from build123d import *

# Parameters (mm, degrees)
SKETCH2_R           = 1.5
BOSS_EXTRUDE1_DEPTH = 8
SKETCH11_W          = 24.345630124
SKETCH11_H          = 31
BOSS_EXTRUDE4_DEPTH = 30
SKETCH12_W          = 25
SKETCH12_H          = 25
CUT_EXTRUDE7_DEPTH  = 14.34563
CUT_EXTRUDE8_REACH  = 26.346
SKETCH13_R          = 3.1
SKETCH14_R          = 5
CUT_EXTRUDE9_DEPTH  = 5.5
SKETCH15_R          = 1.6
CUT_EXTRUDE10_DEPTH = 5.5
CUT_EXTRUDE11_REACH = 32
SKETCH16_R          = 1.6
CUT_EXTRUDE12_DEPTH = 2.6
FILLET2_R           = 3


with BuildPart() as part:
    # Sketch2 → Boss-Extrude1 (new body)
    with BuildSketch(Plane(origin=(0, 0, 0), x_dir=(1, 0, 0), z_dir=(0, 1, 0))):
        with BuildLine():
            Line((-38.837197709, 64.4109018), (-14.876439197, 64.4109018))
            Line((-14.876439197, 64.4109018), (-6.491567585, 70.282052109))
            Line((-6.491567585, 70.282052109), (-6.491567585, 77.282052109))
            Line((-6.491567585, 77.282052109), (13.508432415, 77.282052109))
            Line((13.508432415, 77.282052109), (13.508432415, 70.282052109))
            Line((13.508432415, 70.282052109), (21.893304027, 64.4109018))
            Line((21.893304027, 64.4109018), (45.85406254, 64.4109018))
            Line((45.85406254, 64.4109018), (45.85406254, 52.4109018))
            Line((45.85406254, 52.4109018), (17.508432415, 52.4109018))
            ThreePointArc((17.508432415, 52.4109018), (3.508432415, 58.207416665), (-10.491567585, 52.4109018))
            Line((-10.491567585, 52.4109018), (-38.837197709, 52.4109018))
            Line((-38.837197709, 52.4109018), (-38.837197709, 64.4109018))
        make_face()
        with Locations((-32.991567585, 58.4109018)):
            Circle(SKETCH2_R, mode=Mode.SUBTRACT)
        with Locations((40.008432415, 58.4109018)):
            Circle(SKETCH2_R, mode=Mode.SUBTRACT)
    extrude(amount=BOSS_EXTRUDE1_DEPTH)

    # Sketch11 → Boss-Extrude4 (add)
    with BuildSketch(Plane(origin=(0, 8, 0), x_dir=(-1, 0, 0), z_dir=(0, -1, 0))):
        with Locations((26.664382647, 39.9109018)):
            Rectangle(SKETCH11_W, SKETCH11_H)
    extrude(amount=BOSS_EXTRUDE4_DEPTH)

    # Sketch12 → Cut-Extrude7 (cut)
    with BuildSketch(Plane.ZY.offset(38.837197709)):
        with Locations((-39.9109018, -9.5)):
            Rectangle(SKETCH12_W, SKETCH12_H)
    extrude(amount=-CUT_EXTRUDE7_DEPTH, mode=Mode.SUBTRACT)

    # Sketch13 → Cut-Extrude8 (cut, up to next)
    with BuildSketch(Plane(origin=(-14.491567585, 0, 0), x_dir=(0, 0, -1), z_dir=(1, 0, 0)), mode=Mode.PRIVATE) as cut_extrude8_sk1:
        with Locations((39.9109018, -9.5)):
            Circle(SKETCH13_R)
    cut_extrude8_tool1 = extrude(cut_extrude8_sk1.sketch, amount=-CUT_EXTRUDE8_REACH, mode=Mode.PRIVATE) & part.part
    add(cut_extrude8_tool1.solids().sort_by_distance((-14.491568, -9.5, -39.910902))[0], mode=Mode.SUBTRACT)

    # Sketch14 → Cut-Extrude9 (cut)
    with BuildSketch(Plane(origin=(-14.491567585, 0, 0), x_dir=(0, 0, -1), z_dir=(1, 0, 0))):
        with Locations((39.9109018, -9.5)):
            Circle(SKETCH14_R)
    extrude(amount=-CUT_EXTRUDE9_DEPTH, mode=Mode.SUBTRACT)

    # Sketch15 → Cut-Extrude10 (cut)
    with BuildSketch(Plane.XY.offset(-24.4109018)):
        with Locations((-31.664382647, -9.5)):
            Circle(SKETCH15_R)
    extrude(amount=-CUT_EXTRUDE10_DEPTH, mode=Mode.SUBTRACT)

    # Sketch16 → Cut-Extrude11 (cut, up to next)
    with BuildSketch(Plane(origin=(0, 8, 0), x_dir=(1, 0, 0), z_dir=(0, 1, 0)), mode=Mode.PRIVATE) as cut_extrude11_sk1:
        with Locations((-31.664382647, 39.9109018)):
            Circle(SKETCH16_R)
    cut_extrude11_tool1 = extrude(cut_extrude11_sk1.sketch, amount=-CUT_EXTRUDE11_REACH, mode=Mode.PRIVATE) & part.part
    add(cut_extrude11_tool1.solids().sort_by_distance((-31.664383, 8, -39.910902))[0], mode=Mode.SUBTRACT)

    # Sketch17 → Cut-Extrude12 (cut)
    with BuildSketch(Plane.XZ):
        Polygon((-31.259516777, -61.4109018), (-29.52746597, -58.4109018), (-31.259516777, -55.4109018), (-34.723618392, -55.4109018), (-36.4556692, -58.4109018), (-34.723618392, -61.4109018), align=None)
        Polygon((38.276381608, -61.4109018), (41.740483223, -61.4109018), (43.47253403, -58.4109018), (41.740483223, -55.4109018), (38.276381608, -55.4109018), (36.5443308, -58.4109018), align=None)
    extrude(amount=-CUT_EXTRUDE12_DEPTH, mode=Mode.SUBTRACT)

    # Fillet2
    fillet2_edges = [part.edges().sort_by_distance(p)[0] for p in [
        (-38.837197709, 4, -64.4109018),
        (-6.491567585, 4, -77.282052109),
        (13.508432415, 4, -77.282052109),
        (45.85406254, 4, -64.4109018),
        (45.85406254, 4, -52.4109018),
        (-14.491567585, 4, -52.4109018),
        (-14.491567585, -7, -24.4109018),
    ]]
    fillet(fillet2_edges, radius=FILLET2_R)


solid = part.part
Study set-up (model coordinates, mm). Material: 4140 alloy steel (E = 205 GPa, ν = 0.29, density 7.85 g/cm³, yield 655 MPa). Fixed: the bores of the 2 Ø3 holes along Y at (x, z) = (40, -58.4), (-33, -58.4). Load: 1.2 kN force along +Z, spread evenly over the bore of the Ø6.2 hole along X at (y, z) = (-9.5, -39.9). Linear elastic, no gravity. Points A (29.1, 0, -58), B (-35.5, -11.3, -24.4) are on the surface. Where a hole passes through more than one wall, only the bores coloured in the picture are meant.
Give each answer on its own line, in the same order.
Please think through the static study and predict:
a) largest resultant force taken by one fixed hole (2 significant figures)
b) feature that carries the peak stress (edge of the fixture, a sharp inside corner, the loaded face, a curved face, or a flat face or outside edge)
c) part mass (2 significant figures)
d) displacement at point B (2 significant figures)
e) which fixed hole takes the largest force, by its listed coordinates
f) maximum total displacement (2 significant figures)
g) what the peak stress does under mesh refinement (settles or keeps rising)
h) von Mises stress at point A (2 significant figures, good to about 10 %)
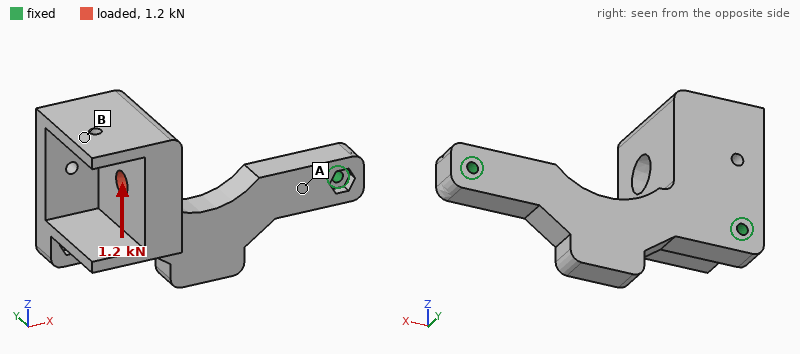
1.1 kN
edge of the fixture
170 g
72 µm
(-33, -58.4)
90 µm
keeps rising
31 MPa
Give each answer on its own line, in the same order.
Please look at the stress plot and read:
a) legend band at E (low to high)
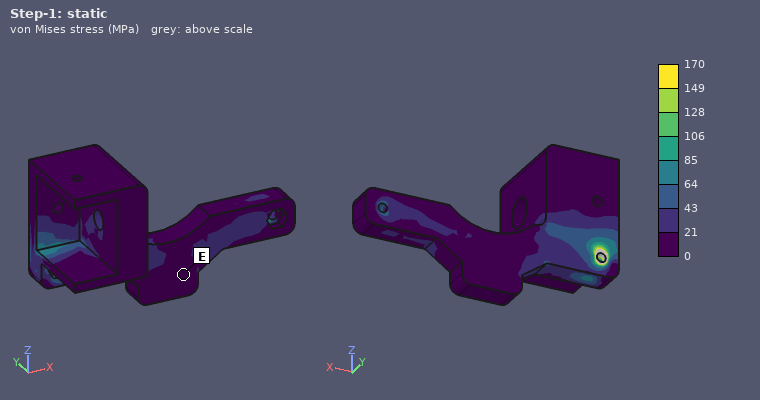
0 to 21 MPa
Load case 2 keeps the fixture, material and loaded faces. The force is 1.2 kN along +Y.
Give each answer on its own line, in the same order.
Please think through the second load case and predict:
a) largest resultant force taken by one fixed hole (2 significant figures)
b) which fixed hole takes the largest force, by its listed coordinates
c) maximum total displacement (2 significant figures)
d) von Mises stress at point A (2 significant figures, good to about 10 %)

1.1 kN
(-33, -58.4)
0.11 mm
32 MPa
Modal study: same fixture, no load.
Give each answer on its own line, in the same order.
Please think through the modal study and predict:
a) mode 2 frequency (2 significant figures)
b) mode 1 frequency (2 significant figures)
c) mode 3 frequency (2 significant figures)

3000 Hz
1900 Hz
4500 Hz
